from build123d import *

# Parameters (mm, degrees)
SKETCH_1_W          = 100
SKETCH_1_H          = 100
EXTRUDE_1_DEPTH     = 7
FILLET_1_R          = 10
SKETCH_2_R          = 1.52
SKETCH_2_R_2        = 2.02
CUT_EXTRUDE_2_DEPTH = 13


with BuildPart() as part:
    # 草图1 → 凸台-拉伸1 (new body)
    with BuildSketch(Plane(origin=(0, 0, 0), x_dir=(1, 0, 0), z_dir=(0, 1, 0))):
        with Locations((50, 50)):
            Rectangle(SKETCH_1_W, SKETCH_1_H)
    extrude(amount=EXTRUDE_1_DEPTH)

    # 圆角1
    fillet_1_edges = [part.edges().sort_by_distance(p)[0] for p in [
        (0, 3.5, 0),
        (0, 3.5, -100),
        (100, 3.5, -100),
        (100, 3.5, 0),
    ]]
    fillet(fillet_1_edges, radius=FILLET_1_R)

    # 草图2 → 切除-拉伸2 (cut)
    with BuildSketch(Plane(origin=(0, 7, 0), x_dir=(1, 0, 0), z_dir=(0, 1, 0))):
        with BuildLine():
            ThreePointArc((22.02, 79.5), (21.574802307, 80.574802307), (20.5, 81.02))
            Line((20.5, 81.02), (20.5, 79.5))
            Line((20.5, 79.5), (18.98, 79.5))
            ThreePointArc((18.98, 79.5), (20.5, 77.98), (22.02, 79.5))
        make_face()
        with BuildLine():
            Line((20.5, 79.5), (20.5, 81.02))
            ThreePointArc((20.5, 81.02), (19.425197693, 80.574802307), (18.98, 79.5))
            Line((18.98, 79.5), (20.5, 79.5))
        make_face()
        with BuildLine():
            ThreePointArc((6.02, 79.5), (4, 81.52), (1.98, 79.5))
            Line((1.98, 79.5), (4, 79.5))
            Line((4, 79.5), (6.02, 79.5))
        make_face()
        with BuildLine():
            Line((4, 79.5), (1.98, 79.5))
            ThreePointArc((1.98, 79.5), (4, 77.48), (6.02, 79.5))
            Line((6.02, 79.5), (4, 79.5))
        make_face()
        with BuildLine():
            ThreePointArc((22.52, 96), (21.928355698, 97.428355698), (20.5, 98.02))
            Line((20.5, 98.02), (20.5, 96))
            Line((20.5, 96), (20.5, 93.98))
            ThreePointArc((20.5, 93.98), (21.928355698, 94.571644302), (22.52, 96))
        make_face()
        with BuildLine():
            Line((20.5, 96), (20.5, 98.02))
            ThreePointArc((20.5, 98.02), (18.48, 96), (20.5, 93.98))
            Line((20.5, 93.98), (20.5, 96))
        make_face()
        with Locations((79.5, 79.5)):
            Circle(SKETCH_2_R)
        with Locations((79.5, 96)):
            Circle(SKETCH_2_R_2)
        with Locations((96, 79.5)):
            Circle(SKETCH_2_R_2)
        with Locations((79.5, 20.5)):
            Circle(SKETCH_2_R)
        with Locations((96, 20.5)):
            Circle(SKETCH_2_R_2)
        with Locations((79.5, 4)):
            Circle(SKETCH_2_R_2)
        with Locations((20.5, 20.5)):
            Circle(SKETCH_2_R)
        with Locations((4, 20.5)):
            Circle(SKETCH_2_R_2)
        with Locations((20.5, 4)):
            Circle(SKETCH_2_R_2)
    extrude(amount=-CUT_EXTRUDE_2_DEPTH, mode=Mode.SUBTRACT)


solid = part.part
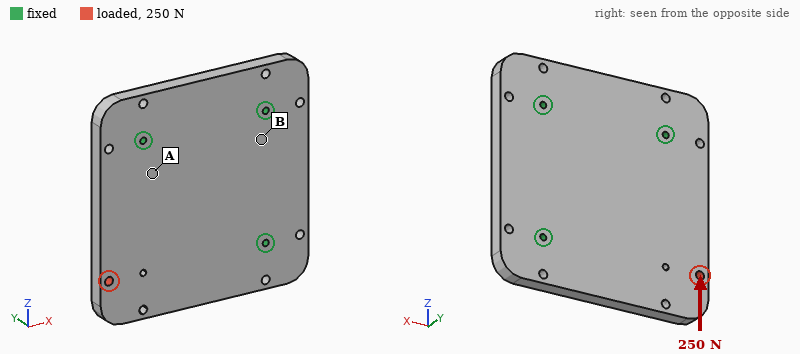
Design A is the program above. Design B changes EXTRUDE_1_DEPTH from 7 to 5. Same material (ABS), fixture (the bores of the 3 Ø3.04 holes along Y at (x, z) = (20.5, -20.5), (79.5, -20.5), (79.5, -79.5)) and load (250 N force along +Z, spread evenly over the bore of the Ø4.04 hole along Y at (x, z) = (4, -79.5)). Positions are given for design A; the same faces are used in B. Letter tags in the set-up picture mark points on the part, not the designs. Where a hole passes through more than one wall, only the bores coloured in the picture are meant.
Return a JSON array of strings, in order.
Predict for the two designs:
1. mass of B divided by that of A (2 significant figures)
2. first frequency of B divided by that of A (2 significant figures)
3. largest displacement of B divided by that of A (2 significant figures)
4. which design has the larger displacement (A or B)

["0.71", "0.74", "1.4", "B"]
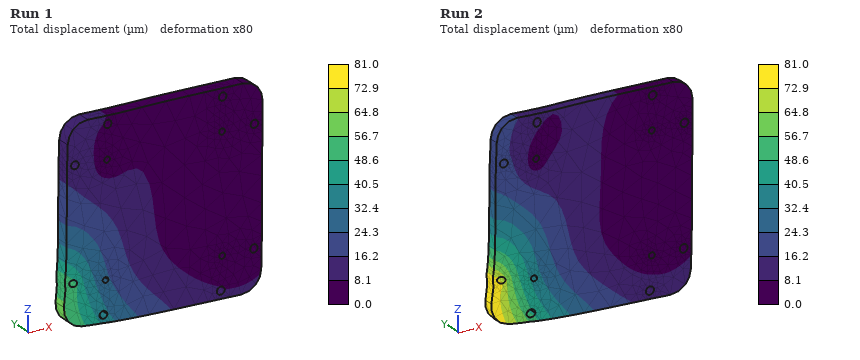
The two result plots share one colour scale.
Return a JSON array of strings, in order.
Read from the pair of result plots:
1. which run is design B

["Run 2"]
